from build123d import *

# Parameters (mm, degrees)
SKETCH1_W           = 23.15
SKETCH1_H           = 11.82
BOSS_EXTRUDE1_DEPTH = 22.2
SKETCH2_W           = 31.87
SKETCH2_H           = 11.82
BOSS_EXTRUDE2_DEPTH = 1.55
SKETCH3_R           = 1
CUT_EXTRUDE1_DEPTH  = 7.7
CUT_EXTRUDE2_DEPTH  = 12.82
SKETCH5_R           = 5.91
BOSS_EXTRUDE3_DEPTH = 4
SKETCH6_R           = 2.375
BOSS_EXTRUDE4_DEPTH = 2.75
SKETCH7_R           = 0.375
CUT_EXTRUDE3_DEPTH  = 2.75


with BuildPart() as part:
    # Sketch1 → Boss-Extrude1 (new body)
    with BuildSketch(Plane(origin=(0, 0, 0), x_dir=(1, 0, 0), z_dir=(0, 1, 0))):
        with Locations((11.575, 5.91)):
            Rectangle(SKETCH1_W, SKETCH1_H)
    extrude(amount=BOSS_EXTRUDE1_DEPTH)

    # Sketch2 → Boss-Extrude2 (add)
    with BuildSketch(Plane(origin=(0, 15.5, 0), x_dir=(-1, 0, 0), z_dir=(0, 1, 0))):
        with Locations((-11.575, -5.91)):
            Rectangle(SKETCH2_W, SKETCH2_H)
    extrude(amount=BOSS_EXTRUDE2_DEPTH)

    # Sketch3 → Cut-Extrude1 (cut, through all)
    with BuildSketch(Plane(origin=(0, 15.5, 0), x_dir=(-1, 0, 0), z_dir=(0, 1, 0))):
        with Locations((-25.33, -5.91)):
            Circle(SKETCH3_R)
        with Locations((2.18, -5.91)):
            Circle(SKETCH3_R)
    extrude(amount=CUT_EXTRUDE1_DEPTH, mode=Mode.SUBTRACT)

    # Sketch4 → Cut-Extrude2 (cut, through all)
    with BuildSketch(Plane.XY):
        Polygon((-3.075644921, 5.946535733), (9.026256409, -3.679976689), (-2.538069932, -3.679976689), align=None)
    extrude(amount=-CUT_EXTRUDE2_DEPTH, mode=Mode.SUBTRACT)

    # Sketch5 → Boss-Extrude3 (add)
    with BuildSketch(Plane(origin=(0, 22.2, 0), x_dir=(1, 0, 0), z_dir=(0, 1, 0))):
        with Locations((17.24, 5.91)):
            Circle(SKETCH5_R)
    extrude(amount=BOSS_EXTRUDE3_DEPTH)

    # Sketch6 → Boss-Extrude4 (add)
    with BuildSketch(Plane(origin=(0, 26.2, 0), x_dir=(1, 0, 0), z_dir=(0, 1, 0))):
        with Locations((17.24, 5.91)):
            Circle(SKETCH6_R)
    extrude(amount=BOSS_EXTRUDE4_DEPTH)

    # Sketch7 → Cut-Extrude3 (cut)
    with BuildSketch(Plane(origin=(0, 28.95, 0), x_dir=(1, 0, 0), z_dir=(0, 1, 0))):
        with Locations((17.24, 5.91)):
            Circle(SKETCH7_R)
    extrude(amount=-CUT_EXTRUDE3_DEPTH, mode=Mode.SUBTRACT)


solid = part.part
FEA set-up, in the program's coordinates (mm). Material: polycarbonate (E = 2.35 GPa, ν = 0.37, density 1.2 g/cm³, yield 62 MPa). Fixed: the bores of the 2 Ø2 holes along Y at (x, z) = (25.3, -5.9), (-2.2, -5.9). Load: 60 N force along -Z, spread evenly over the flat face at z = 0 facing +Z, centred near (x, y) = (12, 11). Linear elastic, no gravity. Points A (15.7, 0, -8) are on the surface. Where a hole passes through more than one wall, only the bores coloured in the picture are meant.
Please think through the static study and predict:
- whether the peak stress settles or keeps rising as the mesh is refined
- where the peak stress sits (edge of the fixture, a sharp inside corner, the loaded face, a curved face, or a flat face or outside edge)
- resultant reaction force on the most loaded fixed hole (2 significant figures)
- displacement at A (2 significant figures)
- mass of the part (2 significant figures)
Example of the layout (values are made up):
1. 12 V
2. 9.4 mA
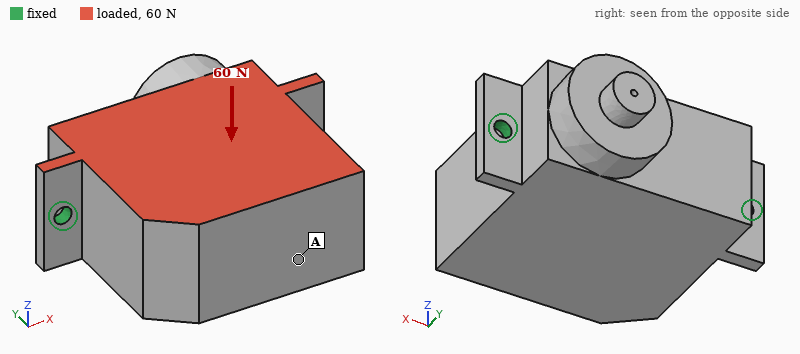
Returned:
1. keeps rising
2. edge of the fixture
3. 30 N
4. 0.39 mm
5. 7.9 g
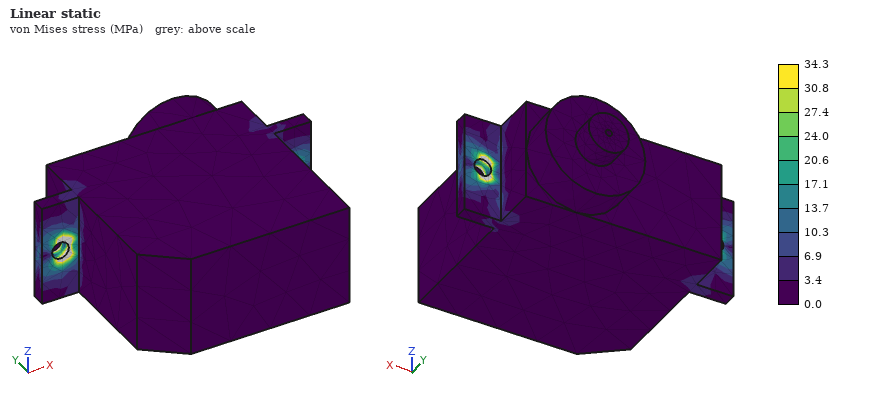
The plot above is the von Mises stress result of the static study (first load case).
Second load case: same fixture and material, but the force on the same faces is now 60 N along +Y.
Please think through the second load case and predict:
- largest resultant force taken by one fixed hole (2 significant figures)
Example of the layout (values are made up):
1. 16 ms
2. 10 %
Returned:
1. 30 N
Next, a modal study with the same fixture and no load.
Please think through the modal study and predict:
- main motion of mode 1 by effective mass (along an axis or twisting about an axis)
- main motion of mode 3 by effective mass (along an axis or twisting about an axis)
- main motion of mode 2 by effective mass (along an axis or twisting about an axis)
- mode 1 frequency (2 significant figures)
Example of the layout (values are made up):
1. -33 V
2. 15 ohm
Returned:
1. along Z
2. along X
3. along Y
4. 730 Hz
